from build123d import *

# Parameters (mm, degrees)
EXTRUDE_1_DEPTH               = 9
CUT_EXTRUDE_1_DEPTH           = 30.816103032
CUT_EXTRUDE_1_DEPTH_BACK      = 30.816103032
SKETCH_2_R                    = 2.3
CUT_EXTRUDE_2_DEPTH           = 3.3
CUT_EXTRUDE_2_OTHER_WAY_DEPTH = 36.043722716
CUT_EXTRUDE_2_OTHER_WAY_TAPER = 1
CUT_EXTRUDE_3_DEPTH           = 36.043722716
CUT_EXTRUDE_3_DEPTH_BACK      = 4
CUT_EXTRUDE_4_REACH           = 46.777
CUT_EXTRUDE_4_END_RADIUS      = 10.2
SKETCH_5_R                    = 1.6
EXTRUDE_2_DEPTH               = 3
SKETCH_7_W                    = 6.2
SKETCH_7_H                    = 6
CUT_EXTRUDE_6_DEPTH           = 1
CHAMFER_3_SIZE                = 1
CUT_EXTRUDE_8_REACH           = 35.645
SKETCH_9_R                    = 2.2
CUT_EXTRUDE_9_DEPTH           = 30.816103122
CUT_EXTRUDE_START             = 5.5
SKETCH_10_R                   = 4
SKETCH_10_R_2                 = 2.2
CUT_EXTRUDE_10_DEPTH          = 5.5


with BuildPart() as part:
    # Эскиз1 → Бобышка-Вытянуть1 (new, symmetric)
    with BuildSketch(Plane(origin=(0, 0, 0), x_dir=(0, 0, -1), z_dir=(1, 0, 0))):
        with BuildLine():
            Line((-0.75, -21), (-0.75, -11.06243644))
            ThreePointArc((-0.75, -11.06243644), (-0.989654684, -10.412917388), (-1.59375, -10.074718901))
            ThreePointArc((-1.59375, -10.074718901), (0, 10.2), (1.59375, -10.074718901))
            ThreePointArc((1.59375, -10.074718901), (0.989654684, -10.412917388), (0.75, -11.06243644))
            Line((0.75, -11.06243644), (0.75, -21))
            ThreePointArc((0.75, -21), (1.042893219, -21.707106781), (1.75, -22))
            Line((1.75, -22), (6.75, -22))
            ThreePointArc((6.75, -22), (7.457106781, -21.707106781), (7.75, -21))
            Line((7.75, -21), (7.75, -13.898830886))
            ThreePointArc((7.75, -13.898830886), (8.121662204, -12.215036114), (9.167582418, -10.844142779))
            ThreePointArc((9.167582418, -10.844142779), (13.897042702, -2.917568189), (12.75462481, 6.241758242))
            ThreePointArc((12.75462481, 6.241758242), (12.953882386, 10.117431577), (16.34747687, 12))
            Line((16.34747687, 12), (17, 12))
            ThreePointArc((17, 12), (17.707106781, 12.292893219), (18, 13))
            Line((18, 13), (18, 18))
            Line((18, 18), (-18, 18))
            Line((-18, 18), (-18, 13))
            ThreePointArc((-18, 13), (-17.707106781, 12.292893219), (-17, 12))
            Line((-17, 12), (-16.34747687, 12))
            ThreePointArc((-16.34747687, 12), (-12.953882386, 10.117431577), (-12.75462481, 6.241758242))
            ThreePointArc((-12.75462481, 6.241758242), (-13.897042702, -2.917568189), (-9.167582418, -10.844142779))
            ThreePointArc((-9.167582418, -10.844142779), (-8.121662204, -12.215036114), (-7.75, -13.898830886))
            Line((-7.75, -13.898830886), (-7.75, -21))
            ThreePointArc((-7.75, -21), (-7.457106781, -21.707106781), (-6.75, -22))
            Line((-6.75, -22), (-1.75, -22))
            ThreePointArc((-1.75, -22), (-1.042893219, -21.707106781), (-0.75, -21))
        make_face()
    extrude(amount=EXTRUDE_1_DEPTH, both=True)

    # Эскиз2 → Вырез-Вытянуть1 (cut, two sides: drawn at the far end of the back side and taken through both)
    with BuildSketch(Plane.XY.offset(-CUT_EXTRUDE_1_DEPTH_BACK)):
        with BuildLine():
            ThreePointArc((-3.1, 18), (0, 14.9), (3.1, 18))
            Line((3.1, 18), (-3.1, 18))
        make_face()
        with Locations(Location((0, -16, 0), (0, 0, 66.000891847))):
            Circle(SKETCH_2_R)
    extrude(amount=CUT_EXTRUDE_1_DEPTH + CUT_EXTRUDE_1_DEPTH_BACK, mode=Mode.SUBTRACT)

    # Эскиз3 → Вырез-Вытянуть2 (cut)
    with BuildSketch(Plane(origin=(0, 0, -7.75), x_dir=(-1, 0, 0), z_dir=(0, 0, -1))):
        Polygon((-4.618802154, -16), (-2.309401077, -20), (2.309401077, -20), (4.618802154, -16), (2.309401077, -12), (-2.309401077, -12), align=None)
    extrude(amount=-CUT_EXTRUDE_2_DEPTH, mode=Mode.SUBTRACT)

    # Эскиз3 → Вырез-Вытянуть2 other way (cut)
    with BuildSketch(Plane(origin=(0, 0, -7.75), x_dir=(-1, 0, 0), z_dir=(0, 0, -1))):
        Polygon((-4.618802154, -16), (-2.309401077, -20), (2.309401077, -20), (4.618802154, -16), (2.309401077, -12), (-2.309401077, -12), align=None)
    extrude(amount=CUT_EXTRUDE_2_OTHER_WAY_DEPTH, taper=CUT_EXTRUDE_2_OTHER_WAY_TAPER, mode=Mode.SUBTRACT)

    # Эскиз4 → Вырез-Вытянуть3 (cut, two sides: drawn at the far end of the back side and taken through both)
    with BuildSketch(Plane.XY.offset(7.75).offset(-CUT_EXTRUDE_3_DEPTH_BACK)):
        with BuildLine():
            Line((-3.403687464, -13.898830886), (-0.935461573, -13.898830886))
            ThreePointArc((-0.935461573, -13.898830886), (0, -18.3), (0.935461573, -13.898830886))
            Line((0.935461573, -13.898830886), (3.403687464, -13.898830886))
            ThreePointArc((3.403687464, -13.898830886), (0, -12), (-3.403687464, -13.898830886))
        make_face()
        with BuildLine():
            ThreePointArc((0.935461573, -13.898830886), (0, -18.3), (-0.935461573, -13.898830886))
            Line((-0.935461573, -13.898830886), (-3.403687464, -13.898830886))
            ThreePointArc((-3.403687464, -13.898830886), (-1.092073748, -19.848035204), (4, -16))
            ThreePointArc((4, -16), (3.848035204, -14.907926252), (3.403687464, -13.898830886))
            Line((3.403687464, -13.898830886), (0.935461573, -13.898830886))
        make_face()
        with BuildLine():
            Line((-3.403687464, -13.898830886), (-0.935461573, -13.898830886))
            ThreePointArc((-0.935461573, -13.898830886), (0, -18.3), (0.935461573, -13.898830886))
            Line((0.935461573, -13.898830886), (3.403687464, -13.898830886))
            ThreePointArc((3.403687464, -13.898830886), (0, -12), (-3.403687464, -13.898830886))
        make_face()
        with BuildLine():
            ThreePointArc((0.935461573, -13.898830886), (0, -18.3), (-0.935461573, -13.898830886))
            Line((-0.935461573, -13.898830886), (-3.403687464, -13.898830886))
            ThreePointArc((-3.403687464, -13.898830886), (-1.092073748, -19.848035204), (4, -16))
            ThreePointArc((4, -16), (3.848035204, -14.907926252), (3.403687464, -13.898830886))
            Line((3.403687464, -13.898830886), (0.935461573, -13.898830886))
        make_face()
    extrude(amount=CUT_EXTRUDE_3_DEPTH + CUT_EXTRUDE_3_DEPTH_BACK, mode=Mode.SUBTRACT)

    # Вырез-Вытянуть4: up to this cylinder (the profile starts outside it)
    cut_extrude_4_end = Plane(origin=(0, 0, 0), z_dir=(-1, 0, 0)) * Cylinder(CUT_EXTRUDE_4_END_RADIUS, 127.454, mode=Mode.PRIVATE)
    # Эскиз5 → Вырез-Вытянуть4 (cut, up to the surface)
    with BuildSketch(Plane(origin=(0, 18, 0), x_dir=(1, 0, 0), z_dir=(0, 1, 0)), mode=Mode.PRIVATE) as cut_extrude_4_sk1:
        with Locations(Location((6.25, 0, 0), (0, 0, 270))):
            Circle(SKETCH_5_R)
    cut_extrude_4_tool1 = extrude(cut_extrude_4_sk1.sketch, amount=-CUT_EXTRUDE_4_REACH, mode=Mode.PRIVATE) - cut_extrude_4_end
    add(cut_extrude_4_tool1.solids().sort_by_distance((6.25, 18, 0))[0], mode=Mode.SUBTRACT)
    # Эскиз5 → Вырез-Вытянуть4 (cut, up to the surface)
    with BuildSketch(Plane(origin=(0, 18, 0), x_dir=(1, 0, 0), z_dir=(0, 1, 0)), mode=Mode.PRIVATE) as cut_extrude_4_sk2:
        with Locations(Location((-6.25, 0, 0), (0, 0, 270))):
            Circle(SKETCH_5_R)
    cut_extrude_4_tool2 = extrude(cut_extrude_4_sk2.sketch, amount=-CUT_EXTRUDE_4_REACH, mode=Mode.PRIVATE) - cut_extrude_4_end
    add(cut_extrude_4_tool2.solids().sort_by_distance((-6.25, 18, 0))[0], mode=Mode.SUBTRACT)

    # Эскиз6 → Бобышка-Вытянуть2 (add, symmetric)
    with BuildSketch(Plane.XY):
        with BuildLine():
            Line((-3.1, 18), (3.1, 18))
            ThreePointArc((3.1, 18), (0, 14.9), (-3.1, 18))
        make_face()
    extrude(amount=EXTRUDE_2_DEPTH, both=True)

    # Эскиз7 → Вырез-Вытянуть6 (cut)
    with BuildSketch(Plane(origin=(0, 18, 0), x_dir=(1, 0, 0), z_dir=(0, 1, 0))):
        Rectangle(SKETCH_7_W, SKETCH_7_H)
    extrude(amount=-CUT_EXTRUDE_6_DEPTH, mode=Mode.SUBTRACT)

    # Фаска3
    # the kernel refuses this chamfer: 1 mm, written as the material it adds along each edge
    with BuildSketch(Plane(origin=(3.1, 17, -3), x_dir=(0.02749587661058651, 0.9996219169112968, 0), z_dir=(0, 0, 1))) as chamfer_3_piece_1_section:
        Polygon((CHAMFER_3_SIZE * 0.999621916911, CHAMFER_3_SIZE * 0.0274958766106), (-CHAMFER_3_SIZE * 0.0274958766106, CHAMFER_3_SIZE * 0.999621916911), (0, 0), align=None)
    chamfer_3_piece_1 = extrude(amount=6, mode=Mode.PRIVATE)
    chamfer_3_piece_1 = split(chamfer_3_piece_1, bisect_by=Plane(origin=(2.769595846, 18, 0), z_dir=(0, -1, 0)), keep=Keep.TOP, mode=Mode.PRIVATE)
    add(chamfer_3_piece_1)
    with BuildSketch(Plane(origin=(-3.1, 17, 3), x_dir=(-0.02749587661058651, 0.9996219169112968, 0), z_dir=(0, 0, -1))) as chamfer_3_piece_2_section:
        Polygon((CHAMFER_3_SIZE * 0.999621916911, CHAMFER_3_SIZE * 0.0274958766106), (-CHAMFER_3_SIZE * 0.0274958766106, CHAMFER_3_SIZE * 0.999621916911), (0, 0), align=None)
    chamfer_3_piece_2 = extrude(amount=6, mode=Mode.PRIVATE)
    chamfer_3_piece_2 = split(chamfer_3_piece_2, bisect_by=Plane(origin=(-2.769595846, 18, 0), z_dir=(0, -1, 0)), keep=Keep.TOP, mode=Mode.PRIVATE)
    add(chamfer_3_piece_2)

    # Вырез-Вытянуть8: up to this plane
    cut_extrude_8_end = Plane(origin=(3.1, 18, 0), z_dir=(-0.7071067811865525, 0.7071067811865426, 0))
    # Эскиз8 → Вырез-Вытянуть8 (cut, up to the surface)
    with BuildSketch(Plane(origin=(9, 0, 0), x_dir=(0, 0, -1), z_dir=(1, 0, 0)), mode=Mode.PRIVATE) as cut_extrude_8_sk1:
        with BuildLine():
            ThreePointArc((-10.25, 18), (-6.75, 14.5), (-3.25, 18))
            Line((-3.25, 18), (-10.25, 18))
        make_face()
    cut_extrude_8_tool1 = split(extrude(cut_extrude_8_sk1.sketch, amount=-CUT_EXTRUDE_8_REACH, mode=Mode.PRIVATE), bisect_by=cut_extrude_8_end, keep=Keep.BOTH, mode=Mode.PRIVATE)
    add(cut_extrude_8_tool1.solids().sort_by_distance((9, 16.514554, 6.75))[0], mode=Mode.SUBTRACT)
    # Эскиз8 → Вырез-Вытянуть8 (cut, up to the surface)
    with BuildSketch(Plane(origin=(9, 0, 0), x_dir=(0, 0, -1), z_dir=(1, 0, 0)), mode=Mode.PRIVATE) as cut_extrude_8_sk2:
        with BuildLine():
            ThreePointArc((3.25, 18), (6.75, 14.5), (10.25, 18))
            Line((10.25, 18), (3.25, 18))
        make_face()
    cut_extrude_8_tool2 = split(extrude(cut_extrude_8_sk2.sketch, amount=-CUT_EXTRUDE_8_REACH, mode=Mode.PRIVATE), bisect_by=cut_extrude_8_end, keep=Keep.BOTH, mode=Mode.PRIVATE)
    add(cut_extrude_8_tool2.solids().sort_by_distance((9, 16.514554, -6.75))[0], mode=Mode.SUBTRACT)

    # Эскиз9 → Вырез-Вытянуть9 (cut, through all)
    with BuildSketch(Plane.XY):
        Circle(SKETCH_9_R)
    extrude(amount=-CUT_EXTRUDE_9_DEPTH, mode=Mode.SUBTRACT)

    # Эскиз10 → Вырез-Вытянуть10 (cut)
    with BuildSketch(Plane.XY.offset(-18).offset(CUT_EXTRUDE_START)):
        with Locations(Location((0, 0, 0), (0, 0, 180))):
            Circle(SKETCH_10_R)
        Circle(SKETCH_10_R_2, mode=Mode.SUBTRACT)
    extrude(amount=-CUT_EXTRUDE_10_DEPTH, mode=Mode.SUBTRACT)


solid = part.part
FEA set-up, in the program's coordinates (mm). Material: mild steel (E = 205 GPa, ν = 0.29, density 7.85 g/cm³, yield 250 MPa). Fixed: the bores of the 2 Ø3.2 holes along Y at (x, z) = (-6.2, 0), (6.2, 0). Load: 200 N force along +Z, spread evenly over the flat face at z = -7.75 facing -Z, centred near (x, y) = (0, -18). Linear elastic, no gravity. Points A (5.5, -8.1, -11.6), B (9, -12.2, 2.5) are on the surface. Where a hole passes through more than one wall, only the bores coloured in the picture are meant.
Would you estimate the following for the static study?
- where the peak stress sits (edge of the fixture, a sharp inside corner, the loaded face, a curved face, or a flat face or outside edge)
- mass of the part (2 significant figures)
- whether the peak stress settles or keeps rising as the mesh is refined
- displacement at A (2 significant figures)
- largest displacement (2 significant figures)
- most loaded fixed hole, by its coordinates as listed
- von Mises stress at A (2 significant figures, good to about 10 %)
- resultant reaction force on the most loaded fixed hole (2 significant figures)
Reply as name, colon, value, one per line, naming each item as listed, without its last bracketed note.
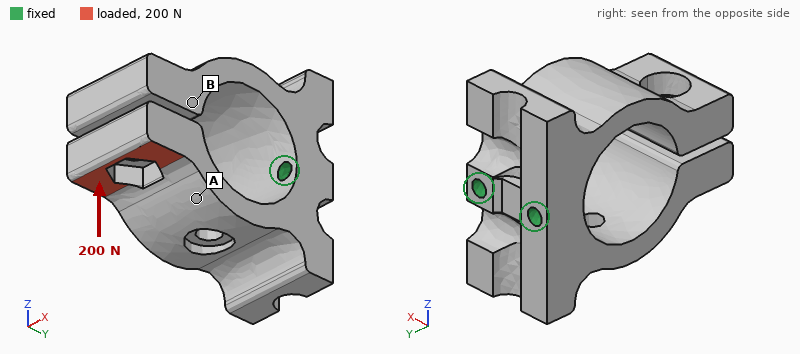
where the peak stress sits: a sharp inside corner
mass of the part: 79 g
whether the peak stress settles or keeps rising as the mesh is refined: keeps rising
displacement at A: 0.046 mm
largest displacement: 0.12 mm
most loaded fixed hole, by its coordinates as listed: (6.2, 0)
von Mises stress at A: 42 MPa
resultant reaction force on the most loaded fixed hole: 120 N
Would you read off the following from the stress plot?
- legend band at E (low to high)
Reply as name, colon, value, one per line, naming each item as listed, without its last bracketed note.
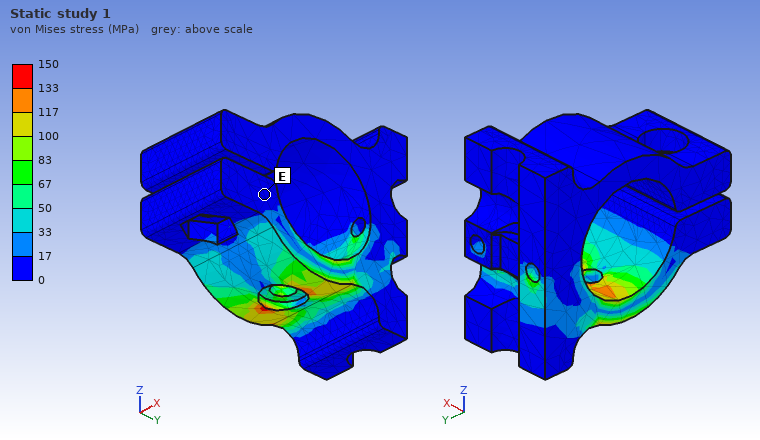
legend band at E: 0 to 17 MPa
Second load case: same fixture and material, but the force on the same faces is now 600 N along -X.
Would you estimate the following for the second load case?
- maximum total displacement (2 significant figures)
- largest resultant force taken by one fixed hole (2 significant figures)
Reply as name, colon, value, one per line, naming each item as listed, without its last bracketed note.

maximum total displacement: 68 µm
largest resultant force taken by one fixed hole: 1.3 kN
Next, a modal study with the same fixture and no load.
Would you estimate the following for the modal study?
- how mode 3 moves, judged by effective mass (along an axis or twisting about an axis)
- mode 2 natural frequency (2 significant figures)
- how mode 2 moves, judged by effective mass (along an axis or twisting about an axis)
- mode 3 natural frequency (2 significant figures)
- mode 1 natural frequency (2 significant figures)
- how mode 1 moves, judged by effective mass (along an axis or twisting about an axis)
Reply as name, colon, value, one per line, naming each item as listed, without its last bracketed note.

how mode 3 moves, judged by effective mass: along X
mode 2 natural frequency: 2500 Hz
how mode 2 moves, judged by effective mass: along Z
mode 3 natural frequency: 4500 Hz
mode 1 natural frequency: 2300 Hz
how mode 1 moves, judged by effective mass: along Z
